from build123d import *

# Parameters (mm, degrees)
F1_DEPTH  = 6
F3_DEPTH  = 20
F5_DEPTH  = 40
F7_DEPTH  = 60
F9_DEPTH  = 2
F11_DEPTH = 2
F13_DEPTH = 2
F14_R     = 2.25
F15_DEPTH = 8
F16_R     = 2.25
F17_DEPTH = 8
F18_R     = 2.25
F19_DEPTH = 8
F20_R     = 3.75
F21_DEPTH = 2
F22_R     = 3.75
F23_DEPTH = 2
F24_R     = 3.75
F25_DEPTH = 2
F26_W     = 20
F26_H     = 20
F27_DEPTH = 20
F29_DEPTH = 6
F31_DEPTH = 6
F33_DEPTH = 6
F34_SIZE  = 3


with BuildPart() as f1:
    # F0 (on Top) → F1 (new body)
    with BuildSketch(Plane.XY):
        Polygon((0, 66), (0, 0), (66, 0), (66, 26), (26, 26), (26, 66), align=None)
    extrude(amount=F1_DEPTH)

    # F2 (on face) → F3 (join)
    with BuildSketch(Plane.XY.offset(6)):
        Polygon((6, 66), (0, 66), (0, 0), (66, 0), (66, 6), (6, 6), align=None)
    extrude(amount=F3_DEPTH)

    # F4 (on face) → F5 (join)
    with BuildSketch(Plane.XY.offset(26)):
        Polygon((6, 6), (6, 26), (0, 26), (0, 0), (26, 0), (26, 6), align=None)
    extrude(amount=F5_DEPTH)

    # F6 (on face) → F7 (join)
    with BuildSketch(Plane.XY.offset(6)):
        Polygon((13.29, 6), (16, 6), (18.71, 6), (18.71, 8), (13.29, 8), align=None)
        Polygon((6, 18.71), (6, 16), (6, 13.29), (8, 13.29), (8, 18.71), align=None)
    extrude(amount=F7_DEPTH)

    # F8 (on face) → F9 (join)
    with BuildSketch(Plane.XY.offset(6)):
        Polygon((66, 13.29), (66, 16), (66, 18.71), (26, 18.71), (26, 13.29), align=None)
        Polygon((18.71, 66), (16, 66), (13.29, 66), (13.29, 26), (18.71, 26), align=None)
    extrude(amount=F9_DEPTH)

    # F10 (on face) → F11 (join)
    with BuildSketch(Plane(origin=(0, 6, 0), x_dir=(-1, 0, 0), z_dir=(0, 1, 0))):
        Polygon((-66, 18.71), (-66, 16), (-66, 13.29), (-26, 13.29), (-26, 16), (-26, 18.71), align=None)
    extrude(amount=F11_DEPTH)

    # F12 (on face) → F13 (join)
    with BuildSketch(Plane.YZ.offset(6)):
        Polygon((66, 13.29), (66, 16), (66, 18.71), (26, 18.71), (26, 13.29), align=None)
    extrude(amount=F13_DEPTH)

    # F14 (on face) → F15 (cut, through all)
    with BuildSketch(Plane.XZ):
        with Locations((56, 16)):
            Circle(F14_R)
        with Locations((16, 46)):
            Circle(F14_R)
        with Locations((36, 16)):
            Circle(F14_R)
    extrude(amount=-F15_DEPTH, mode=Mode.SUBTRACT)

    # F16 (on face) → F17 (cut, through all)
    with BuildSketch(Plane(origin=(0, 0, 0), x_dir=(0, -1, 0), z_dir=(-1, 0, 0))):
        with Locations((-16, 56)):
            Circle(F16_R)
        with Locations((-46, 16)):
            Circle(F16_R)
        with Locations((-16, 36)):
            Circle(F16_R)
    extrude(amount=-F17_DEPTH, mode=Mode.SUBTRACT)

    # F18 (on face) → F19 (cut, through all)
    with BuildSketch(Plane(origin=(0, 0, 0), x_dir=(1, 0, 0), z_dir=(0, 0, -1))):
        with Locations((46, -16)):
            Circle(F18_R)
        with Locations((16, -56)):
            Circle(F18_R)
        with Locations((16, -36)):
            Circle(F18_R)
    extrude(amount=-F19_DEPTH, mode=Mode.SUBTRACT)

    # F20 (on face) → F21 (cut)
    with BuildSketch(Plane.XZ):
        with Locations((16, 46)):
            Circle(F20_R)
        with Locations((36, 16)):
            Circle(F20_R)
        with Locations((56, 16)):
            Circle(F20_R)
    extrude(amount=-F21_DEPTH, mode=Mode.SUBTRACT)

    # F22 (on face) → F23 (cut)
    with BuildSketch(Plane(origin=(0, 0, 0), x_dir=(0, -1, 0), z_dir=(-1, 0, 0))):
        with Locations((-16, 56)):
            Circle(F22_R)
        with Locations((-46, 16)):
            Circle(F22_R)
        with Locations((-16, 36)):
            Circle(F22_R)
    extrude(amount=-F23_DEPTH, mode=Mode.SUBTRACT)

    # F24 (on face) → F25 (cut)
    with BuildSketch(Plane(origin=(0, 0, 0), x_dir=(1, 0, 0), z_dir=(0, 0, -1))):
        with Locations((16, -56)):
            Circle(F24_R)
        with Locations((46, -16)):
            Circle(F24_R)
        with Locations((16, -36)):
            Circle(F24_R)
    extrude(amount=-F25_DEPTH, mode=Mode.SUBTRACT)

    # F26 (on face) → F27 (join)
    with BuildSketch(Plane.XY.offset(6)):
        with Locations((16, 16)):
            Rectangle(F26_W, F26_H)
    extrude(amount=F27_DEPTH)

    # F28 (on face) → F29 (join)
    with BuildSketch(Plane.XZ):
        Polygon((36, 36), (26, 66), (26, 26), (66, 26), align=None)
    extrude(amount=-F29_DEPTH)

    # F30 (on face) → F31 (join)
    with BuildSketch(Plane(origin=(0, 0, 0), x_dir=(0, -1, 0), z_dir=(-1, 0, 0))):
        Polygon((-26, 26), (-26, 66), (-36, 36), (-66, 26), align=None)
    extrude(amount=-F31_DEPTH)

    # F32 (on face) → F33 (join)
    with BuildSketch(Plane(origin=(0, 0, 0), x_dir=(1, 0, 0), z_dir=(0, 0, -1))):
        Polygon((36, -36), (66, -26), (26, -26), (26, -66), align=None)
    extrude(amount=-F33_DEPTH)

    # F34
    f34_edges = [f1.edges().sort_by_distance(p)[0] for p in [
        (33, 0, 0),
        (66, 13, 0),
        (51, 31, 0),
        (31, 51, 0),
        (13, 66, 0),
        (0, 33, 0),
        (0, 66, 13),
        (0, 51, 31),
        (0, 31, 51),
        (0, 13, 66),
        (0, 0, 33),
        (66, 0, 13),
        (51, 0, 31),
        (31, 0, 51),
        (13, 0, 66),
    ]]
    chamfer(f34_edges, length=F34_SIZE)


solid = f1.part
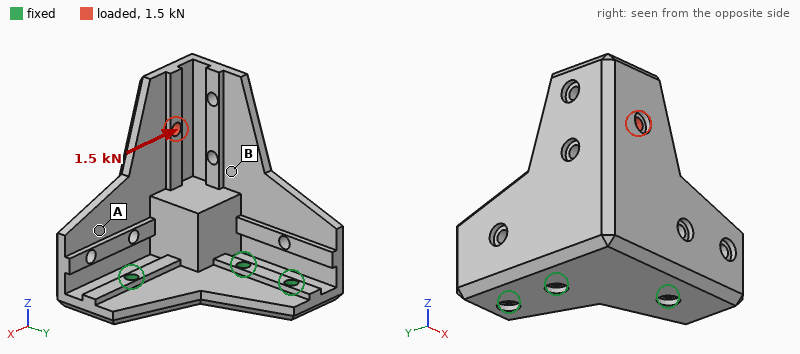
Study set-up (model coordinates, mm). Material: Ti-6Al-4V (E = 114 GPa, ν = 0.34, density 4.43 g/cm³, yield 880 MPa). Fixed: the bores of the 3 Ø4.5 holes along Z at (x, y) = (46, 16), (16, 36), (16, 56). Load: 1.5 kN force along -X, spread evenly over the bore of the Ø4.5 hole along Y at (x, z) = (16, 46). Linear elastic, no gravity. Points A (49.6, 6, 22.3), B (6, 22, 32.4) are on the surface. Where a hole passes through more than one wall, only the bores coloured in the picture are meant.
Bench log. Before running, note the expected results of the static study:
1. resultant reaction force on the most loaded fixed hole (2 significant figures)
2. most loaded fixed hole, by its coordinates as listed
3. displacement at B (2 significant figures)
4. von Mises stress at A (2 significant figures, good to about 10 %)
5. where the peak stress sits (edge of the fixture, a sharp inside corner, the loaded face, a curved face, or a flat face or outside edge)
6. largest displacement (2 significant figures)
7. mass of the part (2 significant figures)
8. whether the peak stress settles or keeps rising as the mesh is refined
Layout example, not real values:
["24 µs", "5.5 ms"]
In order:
["2.3 kN", "(16, 36)", "0.072 mm", "23 MPa", "edge of the fixture", "0.16 mm", "250 g", "keeps rising"]
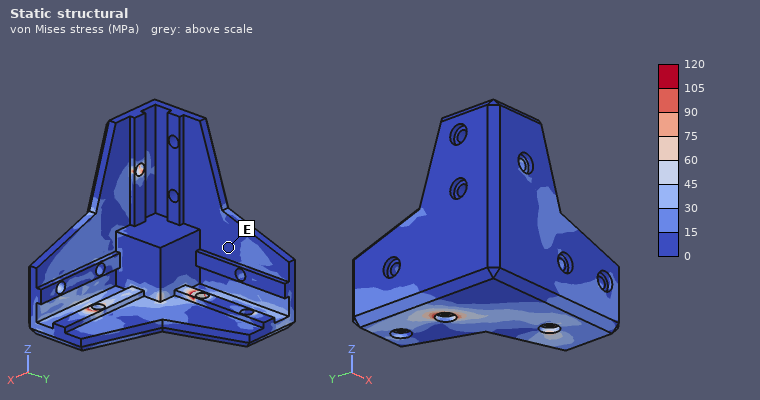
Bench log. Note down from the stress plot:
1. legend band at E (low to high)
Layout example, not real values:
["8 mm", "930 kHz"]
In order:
["0 to 15 MPa"]
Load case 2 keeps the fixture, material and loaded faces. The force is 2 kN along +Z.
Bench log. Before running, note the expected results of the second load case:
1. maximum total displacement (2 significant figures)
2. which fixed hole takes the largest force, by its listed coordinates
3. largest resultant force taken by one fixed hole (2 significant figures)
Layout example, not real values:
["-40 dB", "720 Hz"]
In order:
["0.15 mm", "(16, 36)", "2.8 kN"]
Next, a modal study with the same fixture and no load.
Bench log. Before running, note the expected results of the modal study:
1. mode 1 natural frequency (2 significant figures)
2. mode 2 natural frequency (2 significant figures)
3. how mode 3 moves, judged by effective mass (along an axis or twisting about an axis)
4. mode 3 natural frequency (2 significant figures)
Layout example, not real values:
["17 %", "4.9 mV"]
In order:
["1600 Hz", "3500 Hz", "along Z", "6400 Hz"]
